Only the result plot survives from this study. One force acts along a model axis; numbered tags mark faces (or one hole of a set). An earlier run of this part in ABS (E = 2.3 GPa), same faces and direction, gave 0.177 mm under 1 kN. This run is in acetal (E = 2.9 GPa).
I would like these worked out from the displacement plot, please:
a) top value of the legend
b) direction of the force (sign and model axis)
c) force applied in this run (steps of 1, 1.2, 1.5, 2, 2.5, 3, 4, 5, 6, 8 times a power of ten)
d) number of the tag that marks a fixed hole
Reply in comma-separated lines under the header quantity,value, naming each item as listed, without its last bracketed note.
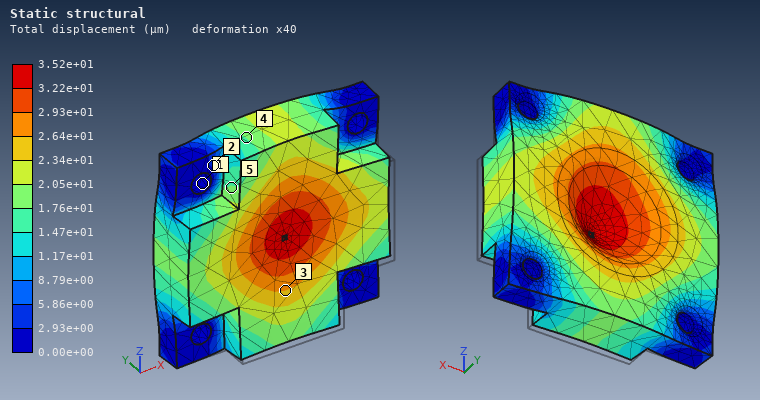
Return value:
quantity,value
top value of the legend,3.52e+01 µm
direction of the force,+Y
force applied in this run,250 N
number of the tag that marks a fixed hole,1
